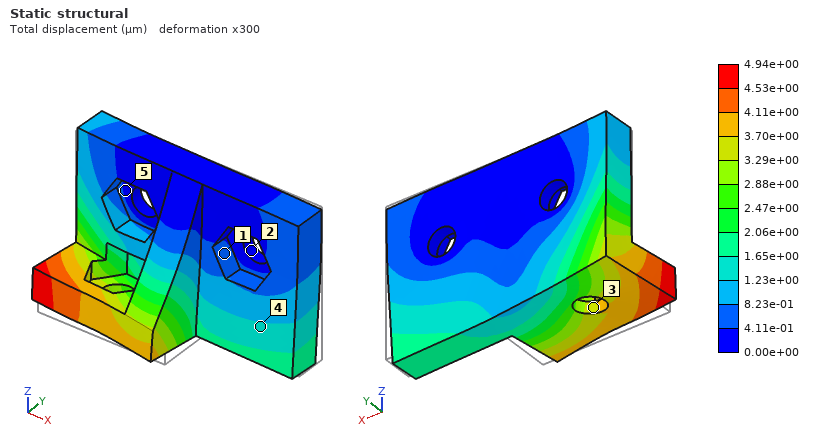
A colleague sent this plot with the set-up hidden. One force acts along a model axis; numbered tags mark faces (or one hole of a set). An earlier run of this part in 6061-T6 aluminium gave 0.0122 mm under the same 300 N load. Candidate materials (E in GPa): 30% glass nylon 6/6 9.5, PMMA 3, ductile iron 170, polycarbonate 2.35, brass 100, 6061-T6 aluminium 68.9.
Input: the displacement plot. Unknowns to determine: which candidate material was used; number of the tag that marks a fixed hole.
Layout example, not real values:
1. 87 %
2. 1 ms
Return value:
1. ductile iron
2. 2
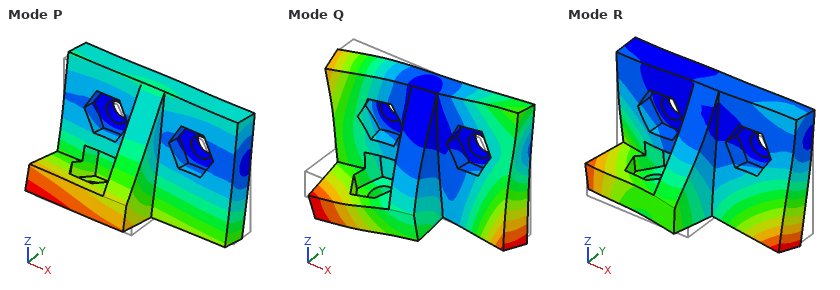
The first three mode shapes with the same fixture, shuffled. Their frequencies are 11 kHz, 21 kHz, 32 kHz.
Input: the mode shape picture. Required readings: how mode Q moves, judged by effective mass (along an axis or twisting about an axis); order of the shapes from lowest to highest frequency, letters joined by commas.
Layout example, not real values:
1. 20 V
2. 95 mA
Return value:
1. along X
2. P, R, Q
